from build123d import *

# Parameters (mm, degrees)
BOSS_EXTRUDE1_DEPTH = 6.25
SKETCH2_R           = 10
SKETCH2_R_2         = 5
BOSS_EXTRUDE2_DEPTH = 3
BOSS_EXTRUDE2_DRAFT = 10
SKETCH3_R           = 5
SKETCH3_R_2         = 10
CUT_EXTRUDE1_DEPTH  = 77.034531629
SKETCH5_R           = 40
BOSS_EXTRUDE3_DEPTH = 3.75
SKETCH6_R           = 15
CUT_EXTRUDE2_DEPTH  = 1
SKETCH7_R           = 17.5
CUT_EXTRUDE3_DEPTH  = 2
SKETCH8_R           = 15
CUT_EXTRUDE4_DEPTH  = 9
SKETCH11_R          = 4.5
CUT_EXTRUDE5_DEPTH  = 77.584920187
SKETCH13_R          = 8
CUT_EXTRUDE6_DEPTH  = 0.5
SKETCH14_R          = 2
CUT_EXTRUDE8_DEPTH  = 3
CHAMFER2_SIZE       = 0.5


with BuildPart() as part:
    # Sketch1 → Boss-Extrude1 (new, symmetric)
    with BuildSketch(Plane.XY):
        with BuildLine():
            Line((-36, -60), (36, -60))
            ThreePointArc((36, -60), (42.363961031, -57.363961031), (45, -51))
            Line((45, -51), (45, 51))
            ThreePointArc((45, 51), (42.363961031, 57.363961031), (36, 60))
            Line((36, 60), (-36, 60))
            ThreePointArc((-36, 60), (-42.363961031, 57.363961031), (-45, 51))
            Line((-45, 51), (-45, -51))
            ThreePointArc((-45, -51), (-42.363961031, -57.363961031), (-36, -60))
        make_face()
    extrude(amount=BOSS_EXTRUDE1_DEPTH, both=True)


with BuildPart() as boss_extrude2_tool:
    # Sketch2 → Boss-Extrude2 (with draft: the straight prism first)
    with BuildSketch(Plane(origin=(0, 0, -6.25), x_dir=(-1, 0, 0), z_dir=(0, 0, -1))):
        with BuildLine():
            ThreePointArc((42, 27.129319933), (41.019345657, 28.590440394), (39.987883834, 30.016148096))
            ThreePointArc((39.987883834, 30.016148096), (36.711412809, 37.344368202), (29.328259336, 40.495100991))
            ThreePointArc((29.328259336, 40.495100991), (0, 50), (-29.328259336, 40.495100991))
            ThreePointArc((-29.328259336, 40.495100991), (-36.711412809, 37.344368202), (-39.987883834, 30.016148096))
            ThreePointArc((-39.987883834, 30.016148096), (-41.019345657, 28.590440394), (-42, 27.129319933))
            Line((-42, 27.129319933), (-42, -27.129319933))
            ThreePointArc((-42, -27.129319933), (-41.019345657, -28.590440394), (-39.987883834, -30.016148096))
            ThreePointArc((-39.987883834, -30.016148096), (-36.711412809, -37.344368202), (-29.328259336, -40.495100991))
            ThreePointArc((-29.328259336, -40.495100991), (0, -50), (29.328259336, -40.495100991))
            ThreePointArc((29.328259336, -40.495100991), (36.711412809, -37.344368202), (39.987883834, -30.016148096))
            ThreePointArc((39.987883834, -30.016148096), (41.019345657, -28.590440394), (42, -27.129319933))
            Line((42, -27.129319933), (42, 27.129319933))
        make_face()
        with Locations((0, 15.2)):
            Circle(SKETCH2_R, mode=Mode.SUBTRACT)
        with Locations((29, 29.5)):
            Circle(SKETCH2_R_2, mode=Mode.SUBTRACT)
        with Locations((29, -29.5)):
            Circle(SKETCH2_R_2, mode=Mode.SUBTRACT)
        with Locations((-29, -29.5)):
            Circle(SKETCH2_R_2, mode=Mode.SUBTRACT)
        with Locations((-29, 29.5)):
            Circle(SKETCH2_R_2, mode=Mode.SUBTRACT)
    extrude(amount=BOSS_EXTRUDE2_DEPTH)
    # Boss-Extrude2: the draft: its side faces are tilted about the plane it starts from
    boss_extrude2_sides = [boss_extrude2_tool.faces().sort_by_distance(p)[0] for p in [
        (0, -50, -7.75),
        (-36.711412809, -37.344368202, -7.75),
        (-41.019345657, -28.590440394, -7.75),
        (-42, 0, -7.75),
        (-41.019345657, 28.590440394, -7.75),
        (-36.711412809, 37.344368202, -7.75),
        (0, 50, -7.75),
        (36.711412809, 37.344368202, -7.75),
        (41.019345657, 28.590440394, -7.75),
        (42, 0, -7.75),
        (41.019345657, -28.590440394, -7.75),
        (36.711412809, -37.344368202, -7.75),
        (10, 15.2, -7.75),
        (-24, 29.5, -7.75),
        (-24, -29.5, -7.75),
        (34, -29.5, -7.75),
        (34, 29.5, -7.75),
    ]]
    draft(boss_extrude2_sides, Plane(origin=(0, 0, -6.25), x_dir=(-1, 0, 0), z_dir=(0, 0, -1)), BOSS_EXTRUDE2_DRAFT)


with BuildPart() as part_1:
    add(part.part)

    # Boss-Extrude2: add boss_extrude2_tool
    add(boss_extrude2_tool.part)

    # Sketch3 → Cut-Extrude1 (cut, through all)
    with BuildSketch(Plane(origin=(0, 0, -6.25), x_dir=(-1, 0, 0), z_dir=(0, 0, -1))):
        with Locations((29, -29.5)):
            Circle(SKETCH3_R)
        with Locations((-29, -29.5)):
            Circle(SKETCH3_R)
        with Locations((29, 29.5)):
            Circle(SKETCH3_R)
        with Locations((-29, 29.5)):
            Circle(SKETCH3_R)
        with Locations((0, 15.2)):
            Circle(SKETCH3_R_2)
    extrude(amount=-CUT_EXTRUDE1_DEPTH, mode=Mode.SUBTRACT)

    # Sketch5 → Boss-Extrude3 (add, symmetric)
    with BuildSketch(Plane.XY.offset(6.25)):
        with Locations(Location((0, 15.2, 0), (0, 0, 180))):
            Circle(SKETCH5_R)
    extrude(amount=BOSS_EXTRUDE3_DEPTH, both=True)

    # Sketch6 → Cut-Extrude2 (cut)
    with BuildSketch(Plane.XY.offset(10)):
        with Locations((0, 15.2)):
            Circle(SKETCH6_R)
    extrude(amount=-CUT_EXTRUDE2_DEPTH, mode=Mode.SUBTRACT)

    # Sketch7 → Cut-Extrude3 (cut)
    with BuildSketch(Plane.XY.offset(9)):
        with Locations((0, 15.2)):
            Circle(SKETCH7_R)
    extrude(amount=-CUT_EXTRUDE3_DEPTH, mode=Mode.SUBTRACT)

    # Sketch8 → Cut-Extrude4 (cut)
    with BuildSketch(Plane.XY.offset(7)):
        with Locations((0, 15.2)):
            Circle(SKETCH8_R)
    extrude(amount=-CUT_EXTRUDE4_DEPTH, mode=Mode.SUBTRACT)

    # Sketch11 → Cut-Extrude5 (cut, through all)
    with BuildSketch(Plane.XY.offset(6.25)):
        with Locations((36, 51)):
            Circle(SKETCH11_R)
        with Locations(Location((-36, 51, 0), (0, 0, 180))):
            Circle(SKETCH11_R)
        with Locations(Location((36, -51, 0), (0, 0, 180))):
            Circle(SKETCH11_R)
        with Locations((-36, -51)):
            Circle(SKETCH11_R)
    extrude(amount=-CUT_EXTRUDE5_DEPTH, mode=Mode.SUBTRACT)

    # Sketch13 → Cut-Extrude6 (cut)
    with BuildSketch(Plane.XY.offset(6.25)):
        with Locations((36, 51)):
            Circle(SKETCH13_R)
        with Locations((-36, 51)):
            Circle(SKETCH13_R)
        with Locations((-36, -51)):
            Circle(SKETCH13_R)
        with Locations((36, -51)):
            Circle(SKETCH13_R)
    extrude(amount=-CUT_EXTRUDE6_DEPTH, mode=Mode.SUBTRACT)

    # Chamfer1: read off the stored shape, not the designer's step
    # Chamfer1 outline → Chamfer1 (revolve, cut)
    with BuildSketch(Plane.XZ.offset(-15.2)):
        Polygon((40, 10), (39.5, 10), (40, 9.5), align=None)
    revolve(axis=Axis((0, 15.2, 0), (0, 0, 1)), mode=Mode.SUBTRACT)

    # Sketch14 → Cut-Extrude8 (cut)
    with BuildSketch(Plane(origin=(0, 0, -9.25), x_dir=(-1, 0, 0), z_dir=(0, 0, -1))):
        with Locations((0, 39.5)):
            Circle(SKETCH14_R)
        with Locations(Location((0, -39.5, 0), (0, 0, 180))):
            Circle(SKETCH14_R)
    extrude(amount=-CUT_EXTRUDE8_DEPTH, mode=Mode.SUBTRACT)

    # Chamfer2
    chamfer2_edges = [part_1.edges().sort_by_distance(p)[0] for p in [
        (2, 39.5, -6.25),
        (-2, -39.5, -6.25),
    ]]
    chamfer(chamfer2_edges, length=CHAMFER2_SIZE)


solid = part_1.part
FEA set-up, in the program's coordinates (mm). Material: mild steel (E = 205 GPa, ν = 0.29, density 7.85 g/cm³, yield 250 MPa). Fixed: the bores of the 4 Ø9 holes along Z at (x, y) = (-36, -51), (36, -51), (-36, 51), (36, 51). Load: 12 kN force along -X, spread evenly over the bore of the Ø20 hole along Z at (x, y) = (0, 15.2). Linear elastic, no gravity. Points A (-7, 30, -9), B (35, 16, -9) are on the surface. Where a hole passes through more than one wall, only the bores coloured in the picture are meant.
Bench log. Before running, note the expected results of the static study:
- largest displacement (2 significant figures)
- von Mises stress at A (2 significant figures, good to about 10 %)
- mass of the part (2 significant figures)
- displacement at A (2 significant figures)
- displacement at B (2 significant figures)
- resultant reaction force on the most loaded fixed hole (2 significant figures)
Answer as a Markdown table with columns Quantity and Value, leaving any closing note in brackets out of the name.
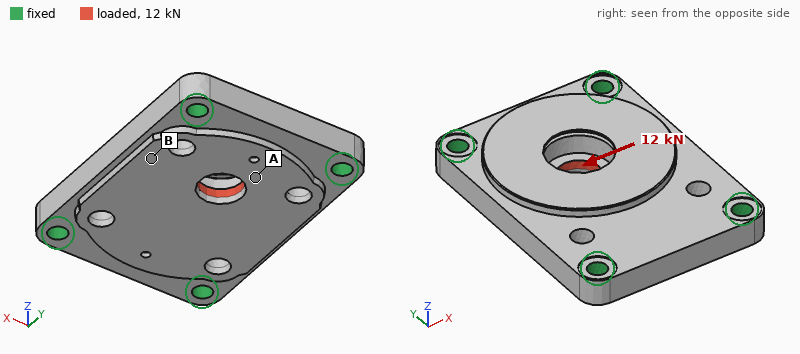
| Quantity | Value |
|---|---|
| largest displacement | 5.7 µm |
| von Mises stress at A | 17 MPa |
| mass of the part | 1.2 kg |
| displacement at A | 2.8 µm |
| displacement at B | 3.8 µm |
| resultant reaction force on the most loaded fixed hole | 4.1 kN |
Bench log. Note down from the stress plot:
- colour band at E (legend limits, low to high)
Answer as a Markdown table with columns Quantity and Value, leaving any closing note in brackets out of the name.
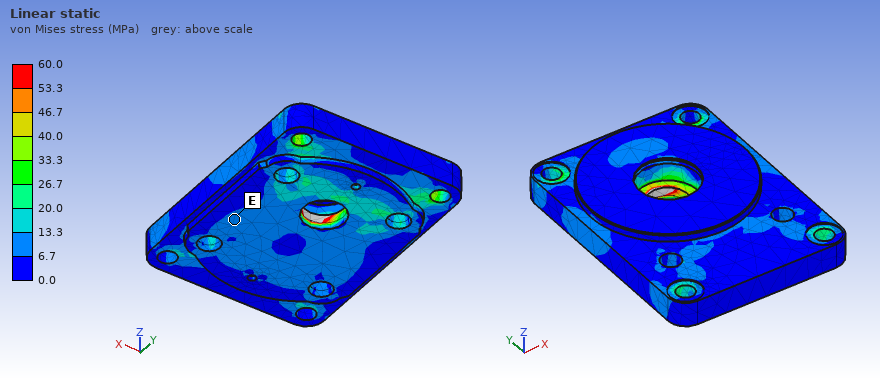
| Quantity | Value |
|---|---|
| colour band at E | 6.7 to 13.3 MPa |
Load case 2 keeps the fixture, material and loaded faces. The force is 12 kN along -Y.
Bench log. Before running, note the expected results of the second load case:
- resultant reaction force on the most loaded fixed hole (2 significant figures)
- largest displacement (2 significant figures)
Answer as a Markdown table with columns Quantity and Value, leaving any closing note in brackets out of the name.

| Quantity | Value |
|---|---|
| resultant reaction force on the most loaded fixed hole | 3.8 kN |
| largest displacement | 4.5 µm |
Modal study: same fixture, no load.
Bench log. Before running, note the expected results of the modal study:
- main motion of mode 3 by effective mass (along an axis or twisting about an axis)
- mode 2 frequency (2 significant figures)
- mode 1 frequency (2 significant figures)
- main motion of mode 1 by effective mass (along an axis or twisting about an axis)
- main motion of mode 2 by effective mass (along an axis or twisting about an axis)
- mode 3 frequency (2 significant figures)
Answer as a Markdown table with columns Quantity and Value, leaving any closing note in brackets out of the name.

| Quantity | Value |
|---|---|
| main motion of mode 3 by effective mass | twisting about X |
| mode 2 frequency | 7700 Hz |
| mode 1 frequency | 5200 Hz |
| main motion of mode 1 by effective mass | along Z |
| main motion of mode 2 by effective mass | twisting about Y |
| mode 3 frequency | 11 kHz |
